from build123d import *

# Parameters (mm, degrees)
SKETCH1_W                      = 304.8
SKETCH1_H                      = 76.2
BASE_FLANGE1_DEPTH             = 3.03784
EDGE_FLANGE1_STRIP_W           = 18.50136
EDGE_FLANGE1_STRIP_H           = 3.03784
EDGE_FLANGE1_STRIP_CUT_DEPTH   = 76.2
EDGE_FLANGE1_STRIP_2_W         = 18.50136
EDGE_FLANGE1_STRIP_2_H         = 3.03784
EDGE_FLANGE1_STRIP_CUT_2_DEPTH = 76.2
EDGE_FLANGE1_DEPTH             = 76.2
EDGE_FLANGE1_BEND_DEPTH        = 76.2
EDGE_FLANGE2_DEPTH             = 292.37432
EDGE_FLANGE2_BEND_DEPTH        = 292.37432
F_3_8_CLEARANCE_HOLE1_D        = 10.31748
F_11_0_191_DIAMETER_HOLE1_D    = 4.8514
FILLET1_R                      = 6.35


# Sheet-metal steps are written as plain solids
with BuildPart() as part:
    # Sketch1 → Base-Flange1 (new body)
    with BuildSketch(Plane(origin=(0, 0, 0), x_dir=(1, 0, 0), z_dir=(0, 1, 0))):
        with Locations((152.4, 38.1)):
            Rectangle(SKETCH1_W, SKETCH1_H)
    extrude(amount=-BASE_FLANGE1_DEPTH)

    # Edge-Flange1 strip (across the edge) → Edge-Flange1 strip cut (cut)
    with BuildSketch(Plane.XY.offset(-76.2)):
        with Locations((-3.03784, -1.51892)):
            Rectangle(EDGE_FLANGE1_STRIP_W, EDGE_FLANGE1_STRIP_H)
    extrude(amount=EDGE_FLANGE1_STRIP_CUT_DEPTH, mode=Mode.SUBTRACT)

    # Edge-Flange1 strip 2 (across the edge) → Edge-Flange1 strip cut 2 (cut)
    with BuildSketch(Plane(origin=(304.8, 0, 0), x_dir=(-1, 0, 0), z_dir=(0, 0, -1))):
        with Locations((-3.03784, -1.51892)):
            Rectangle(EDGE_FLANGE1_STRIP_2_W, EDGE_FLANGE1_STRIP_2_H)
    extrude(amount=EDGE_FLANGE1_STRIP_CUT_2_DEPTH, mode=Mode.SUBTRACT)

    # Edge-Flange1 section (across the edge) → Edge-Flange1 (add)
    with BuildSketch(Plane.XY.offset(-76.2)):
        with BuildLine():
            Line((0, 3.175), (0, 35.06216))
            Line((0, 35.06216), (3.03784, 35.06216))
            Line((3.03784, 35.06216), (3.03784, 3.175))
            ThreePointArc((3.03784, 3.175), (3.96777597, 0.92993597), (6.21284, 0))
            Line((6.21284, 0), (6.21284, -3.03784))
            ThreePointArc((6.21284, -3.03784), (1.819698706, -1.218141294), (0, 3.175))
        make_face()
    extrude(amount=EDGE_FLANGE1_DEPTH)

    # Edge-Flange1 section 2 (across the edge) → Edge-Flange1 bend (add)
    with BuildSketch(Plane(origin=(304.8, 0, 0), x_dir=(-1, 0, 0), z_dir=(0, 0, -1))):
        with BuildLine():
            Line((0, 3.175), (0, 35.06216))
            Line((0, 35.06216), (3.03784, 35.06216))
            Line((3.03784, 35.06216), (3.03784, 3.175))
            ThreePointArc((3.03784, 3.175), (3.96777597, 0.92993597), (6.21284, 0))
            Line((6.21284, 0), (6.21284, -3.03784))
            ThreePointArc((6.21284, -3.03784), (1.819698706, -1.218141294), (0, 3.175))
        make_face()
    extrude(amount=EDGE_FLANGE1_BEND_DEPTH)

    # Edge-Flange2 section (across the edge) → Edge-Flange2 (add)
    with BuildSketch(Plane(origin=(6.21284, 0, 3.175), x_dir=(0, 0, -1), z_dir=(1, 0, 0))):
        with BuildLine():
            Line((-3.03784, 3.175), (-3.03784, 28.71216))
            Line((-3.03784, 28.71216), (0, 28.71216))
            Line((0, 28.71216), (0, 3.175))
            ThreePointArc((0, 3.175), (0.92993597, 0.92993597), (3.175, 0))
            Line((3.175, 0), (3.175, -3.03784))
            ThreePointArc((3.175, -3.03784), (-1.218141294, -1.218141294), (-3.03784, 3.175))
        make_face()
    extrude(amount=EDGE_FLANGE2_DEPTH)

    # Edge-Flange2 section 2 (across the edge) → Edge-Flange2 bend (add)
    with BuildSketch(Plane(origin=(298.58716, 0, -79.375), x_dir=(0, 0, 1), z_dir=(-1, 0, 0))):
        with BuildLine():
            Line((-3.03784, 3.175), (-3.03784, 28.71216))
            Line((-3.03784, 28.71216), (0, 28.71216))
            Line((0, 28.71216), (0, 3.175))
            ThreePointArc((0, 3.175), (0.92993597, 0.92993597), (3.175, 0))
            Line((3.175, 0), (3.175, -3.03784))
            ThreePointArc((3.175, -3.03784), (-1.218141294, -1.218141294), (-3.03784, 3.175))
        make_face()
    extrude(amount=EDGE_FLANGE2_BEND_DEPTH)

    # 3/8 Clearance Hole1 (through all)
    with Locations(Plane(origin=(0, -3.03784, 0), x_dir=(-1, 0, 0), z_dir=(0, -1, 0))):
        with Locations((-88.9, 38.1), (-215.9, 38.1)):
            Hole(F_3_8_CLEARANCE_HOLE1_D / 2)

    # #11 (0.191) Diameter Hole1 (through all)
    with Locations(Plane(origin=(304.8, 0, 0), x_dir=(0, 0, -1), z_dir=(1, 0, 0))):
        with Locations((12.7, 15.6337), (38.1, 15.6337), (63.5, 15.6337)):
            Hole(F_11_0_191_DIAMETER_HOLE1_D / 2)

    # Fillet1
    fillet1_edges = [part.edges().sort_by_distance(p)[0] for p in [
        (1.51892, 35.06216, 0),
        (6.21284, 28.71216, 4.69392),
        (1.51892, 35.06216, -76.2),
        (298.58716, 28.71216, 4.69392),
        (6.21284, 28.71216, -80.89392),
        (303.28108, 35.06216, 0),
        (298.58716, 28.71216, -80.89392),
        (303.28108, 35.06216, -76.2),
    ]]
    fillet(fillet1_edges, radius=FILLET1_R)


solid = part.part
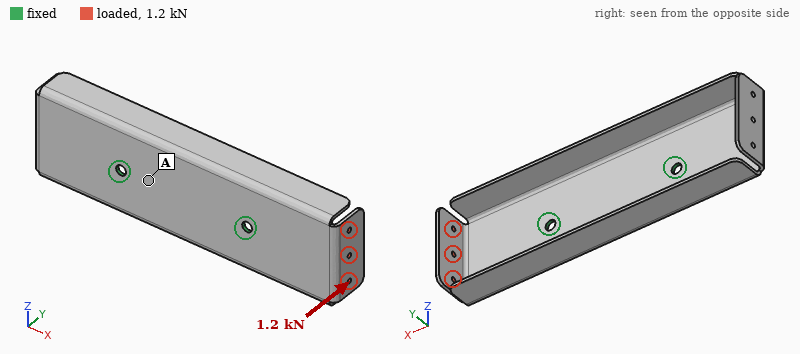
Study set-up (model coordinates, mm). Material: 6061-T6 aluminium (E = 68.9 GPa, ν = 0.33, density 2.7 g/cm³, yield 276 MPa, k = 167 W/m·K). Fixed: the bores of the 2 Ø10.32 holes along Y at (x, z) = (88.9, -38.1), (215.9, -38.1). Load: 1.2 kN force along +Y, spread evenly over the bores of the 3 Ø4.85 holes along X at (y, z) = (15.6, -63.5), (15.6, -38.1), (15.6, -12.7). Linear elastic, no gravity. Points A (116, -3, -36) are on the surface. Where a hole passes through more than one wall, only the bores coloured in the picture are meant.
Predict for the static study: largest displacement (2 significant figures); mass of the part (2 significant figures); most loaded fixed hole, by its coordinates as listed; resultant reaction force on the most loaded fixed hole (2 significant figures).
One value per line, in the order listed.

2.4 mm
390 g
(215.9, -38.1)
2.3 kN
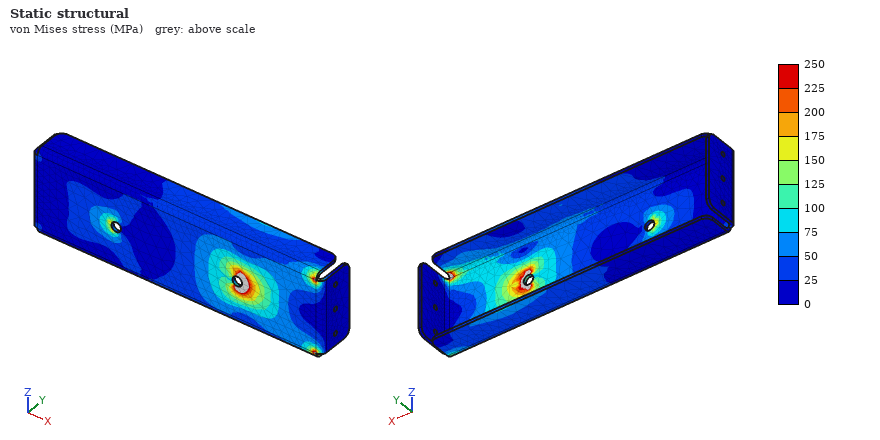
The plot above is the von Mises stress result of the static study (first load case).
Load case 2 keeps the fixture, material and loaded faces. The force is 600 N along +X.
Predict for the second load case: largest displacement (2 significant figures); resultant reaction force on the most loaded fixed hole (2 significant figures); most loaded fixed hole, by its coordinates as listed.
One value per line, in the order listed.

0.73 mm
340 N
(215.9, -38.1)
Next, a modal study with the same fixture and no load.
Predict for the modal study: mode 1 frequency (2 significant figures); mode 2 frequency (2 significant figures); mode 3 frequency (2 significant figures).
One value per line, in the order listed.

380 Hz
390 Hz
400 Hz
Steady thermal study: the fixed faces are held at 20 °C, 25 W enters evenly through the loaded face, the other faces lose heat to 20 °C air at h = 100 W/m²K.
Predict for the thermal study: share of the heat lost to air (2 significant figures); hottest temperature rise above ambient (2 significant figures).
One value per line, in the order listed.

90 %
23 K
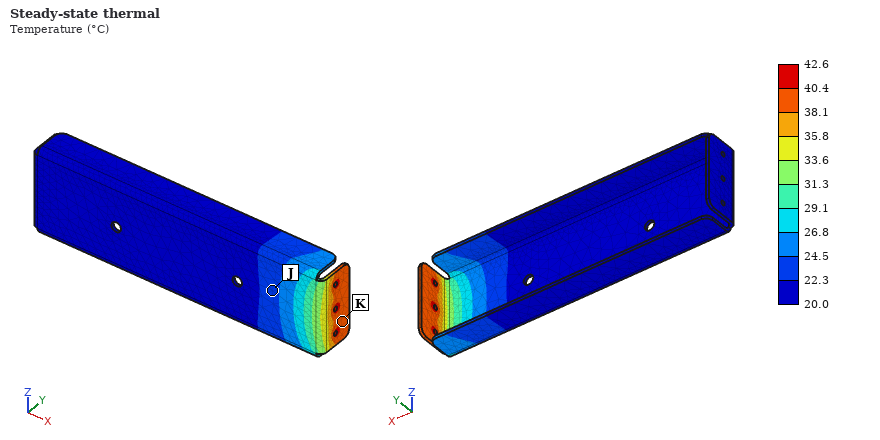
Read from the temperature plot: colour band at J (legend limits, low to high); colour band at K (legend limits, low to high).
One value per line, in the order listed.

22.3 to 24.5 °C
38.1 to 40.4 °C
